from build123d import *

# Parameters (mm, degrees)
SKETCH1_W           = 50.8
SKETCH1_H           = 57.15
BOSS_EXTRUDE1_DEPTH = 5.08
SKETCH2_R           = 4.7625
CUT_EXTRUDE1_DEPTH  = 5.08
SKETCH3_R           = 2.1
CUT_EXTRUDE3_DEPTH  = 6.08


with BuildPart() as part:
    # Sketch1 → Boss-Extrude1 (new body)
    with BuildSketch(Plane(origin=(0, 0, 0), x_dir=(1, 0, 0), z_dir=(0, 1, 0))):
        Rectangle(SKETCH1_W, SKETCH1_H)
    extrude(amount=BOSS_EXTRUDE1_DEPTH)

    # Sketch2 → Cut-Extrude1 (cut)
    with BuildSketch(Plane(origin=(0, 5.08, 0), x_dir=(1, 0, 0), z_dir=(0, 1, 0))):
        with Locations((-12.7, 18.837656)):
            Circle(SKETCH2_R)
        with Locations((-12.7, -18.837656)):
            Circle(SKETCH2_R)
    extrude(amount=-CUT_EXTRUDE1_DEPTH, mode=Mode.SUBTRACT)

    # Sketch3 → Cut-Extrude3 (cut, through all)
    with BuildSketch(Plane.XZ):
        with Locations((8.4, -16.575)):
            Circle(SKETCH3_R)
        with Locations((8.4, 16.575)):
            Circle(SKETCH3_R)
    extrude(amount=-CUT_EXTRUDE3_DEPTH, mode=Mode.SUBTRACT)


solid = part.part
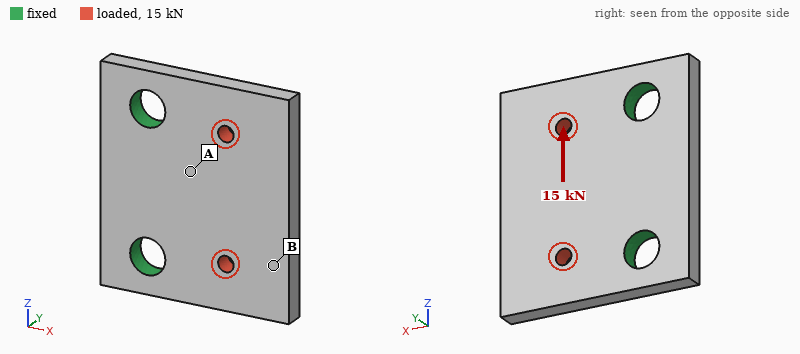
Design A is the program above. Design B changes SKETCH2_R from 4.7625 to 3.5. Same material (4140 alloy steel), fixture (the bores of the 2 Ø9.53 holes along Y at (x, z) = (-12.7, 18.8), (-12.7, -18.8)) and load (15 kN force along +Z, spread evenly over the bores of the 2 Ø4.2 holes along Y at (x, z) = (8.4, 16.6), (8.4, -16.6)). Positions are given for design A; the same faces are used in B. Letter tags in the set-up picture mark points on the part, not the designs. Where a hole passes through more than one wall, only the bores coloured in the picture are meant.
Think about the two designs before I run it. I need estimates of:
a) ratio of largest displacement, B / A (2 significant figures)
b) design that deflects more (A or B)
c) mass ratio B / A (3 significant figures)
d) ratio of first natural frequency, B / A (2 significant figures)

1.2
B
1.02
0.91
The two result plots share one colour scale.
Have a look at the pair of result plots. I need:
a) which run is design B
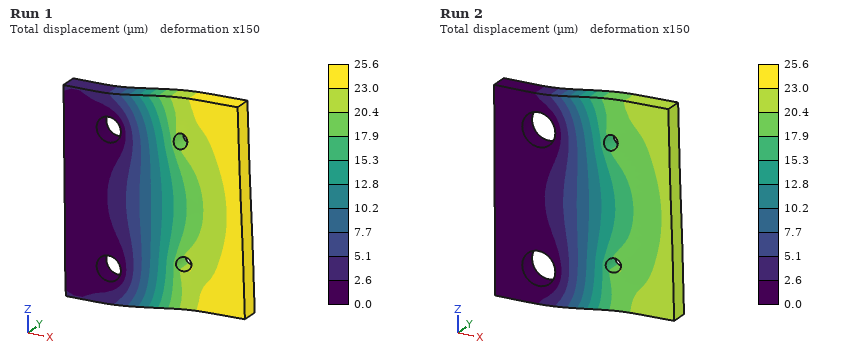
Run 1
